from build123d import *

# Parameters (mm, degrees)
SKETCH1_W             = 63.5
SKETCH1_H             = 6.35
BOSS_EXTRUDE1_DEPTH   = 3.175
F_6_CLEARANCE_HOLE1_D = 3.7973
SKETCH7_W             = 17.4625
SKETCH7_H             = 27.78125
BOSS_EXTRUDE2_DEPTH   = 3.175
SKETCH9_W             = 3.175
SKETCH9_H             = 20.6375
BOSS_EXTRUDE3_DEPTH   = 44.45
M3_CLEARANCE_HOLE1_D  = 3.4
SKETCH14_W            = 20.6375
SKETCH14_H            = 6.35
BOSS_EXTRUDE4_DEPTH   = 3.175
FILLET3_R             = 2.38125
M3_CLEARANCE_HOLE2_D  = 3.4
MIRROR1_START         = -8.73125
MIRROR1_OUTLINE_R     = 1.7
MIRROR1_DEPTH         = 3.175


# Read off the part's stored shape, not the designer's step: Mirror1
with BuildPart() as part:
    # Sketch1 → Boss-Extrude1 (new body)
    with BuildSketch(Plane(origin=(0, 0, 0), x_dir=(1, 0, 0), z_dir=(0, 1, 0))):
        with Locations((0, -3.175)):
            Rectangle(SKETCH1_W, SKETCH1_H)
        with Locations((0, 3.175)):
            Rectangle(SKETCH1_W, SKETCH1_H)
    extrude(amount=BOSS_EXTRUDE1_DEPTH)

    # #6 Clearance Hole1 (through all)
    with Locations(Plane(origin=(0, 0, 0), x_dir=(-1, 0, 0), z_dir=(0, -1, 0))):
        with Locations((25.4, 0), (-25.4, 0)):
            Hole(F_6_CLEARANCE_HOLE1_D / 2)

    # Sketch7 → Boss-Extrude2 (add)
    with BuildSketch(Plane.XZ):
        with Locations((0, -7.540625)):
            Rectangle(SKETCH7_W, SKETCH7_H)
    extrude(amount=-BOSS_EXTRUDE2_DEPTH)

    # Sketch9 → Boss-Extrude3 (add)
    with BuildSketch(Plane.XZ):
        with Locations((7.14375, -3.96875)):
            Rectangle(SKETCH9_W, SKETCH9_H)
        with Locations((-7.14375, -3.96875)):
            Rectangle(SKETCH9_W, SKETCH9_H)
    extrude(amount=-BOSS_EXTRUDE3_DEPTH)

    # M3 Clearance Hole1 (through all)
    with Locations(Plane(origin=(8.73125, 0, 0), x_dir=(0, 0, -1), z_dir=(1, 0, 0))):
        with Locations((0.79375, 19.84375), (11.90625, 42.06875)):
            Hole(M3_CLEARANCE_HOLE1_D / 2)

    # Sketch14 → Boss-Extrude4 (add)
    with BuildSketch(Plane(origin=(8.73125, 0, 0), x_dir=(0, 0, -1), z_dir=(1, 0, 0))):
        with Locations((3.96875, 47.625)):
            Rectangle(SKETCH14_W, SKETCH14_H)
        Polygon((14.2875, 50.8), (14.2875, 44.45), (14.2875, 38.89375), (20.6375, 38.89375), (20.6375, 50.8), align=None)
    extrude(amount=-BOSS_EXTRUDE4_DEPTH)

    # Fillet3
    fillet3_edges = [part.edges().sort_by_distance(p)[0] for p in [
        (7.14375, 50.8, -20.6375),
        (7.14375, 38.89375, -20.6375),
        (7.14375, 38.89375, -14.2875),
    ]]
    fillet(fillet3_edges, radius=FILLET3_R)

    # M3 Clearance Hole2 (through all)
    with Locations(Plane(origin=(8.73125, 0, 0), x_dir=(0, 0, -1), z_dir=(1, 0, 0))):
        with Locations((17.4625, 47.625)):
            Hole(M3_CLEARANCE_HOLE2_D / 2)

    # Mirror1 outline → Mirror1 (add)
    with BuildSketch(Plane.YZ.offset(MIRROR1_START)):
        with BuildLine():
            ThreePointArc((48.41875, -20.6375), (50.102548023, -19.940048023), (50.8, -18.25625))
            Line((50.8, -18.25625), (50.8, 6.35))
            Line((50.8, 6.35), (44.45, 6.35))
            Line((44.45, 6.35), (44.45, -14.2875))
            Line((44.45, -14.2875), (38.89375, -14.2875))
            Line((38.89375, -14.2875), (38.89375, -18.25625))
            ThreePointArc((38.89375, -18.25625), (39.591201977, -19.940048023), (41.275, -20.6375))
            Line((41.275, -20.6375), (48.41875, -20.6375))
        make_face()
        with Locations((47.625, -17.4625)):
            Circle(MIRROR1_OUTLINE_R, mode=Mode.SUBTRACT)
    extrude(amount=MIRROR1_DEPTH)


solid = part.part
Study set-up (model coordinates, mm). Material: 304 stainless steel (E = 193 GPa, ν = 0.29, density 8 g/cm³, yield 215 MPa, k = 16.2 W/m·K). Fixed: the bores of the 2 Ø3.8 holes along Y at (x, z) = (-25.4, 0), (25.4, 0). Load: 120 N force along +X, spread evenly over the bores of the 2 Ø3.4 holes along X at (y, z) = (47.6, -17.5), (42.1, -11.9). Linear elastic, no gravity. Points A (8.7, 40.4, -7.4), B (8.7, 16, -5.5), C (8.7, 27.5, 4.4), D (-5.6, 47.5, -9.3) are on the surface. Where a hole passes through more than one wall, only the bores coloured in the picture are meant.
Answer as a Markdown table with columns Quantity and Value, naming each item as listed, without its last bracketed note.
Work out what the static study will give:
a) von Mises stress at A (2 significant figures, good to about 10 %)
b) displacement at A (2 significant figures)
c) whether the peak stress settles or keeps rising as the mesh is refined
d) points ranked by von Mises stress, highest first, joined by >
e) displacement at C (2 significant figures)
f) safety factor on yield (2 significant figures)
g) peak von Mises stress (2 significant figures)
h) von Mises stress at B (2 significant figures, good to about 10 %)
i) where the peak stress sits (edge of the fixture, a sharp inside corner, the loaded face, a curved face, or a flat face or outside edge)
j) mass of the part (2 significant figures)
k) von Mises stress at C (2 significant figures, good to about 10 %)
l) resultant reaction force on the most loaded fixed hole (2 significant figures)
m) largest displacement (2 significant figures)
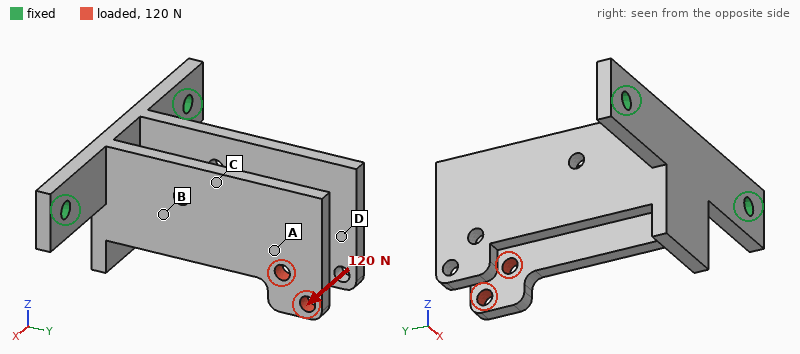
| Quantity | Value |
|---|---|
| von Mises stress at A | 33 MPa |
| displacement at A | 0.32 mm |
| whether the peak stress settles or keeps rising as the mesh is refined | settles |
| points ranked by von Mises stress, highest first, joined by > | B > C > A > D |
| displacement at C | 0.15 mm |
| safety factor on yield | 1.2 |
| peak von Mises stress | 180 MPa |
| von Mises stress at B | 110 MPa |
| where the peak stress sits | a curved face |
| mass of the part | 79 g |
| von Mises stress at C | 66 MPa |
| resultant reaction force on the most loaded fixed hole | 160 N |
| largest displacement | 0.49 mm |
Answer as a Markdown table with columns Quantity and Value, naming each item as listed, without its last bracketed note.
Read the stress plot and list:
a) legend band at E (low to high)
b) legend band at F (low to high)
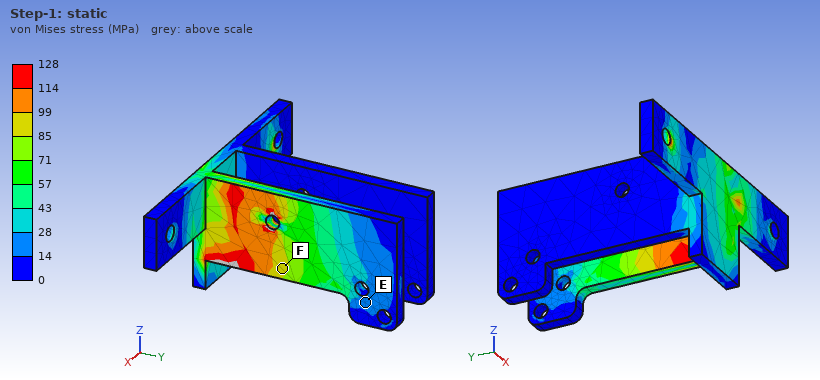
| Quantity | Value |
|---|---|
| legend band at E | 14 to 28 MPa |
| legend band at F | 85 to 99 MPa |
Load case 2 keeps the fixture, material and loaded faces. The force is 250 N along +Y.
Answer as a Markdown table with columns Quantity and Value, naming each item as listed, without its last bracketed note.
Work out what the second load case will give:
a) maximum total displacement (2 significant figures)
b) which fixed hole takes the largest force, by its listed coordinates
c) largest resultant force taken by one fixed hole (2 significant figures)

| Quantity | Value |
|---|---|
| maximum total displacement | 0.19 mm |
| which fixed hole takes the largest force, by its listed coordinates | (25.4, 0) |
| largest resultant force taken by one fixed hole | 180 N |
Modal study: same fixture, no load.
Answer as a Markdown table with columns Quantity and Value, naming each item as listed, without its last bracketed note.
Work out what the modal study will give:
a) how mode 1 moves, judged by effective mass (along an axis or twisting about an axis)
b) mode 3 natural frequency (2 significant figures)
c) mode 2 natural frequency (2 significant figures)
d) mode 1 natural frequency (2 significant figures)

| Quantity | Value |
|---|---|
| how mode 1 moves, judged by effective mass | along Z |
| mode 3 natural frequency | 890 Hz |
| mode 2 natural frequency | 850 Hz |
| mode 1 natural frequency | 750 Hz |
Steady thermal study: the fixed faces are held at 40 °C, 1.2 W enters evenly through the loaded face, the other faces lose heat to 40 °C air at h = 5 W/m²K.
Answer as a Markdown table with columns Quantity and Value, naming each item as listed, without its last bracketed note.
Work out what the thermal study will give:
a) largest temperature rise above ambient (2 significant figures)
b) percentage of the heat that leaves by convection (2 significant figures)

| Quantity | Value |
|---|---|
| largest temperature rise above ambient | 61 K |
| percentage of the heat that leaves by convection | 46 % |
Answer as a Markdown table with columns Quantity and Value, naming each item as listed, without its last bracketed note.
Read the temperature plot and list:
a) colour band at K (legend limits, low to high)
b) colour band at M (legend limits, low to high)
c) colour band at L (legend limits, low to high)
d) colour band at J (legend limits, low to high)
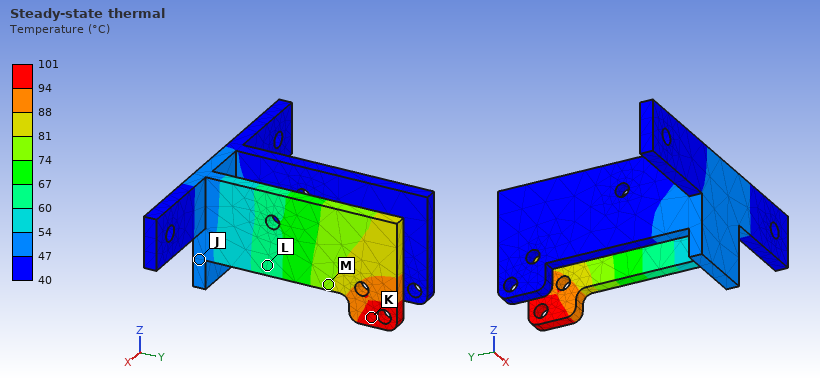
| Quantity | Value |
|---|---|
| colour band at K | 94 to 101 °C |
| colour band at M | 74 to 81 °C |
| colour band at L | 60 to 67 °C |
| colour band at J | 47 to 54 °C |
